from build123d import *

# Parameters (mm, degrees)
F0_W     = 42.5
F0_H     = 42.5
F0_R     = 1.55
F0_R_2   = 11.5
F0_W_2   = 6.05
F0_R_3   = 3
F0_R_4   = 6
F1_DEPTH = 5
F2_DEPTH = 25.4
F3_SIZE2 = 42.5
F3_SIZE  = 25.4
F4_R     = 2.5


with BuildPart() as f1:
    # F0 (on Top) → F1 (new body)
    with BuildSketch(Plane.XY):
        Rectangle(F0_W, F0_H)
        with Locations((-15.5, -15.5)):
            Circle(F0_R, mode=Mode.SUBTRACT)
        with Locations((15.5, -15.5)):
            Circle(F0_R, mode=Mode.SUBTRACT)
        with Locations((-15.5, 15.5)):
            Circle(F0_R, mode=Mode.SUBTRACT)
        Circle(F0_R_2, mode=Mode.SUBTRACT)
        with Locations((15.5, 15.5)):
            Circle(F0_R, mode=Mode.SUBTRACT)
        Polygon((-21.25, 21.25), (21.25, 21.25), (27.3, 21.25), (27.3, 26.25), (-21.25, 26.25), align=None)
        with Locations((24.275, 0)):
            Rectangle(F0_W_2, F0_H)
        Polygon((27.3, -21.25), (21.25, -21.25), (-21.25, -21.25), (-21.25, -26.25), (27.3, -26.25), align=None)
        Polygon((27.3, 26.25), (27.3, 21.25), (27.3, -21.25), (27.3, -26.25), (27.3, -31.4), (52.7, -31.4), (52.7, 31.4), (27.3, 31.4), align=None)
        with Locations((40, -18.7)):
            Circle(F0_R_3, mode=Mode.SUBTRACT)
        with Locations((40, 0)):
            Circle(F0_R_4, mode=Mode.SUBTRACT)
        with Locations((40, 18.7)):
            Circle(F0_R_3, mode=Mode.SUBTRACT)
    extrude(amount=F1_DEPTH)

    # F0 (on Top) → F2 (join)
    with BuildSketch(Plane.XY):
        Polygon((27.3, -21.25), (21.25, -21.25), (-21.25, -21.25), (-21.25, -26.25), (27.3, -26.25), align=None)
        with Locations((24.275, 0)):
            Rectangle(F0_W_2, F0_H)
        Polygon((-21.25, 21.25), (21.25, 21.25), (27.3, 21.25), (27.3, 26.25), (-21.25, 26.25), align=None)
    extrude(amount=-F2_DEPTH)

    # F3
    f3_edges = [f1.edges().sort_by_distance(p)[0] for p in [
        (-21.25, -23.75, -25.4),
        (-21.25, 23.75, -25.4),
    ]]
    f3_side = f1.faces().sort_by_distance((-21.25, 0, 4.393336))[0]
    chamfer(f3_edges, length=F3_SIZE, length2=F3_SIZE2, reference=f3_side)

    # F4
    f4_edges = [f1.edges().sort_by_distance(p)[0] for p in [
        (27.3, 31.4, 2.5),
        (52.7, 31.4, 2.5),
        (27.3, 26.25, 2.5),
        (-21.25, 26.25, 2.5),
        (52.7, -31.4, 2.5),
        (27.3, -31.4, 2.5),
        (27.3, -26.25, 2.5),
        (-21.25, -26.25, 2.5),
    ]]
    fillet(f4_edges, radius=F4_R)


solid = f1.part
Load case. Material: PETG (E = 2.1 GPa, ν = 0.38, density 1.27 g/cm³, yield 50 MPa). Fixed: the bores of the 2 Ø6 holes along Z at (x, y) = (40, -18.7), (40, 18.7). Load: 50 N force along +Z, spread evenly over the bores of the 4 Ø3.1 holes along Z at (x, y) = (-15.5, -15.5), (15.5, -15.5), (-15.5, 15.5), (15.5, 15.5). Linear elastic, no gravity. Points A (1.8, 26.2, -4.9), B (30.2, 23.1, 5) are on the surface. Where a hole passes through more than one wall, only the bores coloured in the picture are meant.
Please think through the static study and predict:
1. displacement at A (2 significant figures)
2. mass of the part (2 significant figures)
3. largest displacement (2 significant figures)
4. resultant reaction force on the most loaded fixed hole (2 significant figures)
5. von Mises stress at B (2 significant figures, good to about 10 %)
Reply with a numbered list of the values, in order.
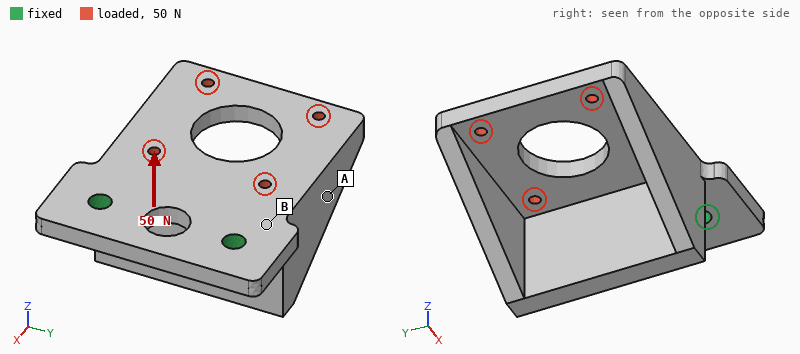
1. 0.64 mm
2. 39 g
3. 1.2 mm
4. 25 N
5. 6.6 MPa
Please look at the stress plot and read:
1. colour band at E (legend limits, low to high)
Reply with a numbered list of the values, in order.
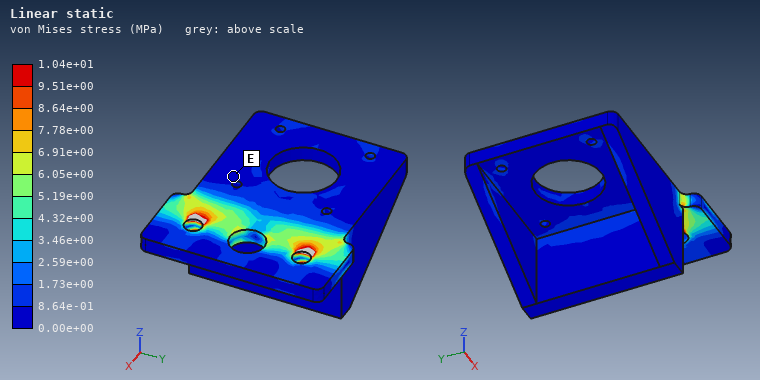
1. 0.00e+00 to 8.64e-01 MPa
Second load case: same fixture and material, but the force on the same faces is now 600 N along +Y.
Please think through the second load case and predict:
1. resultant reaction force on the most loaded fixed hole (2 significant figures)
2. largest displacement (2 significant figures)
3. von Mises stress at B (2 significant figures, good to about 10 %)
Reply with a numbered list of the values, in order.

1. 650 N
2. 0.47 mm
3. 4.5 MPa
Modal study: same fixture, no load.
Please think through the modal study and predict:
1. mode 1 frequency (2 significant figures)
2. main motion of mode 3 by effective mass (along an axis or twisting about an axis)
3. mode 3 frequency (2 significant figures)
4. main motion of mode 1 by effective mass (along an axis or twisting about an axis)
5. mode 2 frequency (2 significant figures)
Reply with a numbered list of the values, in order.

1. 290 Hz
2. along Y
3. 1600 Hz
4. along Z
5. 780 Hz
